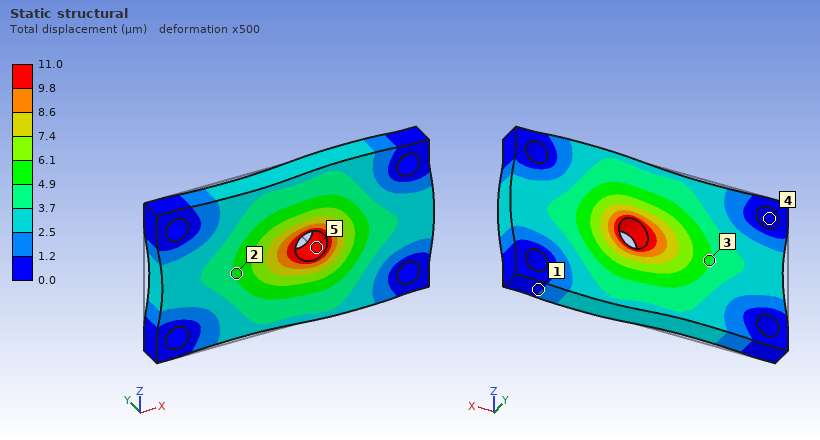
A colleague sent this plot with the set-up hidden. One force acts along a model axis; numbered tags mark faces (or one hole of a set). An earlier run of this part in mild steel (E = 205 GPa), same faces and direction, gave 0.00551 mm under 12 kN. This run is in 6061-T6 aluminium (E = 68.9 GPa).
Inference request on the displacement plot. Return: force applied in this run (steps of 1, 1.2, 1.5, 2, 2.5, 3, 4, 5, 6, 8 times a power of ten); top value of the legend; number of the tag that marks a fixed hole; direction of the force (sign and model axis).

8 kN
11.0 µm
4
+X
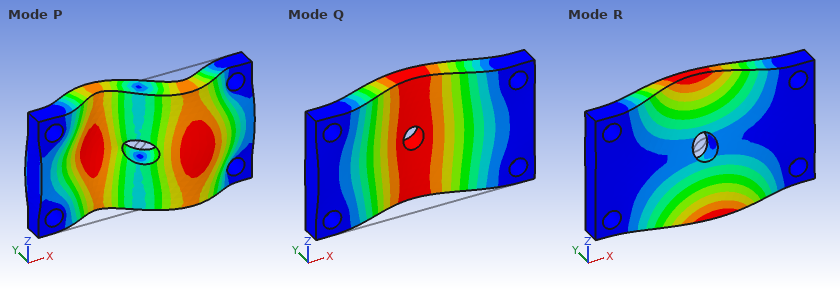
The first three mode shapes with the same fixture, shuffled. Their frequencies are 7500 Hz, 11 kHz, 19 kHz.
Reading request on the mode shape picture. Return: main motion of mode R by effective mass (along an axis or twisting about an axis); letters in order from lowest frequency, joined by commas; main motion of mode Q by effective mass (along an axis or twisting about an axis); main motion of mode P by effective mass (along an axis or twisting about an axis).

twisting about X
Q, R, P
along Y
twisting about Z
